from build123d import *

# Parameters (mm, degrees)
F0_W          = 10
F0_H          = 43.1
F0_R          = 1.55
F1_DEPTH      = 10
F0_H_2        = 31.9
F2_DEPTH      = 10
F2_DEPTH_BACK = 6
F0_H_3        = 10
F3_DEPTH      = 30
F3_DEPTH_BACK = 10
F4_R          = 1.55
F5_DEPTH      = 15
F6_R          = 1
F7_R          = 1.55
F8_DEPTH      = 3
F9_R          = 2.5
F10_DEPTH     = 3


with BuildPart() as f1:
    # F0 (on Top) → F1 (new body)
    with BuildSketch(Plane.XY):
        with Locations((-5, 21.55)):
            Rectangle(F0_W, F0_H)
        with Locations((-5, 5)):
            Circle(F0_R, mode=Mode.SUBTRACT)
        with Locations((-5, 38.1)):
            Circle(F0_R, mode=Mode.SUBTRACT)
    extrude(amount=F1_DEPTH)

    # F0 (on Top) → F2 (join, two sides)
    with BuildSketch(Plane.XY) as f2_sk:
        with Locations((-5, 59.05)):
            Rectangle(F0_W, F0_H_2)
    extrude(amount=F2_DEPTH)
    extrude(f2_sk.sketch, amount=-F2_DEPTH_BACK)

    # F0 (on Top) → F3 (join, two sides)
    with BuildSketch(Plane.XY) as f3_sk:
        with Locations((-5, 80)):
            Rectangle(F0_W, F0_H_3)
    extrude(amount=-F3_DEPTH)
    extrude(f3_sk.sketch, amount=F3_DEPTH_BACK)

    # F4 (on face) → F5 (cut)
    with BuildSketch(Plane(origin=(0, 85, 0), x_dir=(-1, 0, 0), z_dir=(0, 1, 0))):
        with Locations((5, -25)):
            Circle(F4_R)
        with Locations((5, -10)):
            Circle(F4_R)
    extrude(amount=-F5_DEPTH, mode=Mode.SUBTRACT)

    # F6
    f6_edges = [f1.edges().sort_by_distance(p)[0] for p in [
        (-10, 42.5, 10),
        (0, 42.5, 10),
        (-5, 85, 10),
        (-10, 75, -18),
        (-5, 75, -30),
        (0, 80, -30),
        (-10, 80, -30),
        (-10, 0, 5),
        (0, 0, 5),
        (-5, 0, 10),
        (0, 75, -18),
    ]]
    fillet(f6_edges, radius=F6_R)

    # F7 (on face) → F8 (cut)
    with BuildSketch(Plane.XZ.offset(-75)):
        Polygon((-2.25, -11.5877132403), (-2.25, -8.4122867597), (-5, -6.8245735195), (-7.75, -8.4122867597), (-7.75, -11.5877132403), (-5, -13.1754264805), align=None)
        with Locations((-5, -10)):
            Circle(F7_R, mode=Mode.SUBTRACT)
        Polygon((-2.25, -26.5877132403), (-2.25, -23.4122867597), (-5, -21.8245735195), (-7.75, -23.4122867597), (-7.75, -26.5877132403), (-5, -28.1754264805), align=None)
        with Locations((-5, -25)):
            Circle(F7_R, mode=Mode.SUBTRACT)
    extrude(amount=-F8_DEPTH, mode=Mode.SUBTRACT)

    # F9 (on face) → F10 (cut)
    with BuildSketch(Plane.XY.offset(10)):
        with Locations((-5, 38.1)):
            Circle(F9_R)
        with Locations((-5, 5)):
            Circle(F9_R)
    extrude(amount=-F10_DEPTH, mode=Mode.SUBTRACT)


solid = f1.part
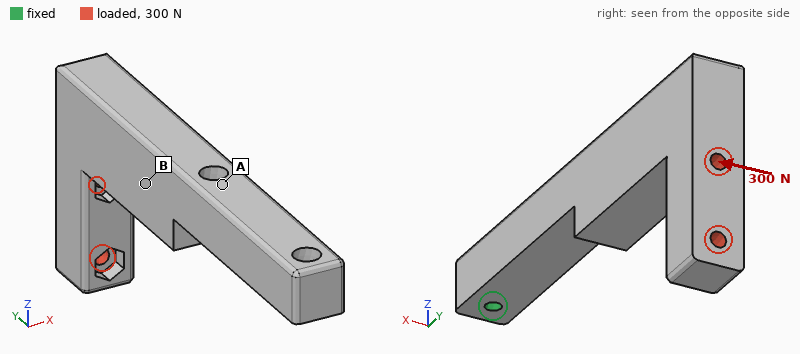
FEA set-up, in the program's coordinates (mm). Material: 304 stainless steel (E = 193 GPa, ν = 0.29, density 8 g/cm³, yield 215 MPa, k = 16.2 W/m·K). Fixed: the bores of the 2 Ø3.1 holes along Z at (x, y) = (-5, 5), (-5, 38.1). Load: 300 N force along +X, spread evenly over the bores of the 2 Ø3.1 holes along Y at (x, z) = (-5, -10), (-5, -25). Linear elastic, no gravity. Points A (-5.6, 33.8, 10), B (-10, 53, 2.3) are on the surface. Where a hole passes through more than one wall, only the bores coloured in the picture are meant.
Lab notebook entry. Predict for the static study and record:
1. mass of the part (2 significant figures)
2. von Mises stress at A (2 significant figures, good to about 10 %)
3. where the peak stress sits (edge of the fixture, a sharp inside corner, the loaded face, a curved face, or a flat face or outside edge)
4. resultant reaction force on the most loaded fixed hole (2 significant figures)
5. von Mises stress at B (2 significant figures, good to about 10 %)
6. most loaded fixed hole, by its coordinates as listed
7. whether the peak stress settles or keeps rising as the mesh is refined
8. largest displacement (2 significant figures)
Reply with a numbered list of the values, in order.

1. 100 g
2. 20 MPa
3. edge of the fixture
4. 510 N
5. 45 MPa
6. (-5, 38.1)
7. keeps rising
8. 0.12 mm
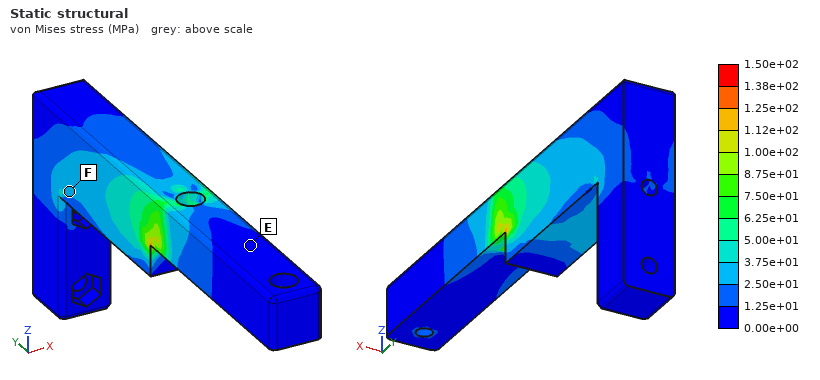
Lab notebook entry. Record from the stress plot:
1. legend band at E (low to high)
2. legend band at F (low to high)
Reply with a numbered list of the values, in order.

1. 0.00e+00 to 1.25e+01 MPa
2. 2.50e+01 to 3.75e+01 MPa
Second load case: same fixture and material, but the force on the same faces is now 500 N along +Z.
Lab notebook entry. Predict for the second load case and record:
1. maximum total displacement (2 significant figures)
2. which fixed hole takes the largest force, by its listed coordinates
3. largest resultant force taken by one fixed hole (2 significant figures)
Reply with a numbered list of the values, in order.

1. 0.11 mm
2. (-5, 38.1)
3. 780 N
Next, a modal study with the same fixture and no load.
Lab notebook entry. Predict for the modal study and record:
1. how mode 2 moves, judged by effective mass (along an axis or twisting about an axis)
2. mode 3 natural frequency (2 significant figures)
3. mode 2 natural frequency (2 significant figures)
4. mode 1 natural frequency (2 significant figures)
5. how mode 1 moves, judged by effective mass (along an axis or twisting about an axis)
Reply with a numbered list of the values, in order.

1. along Z
2. 4500 Hz
3. 2000 Hz
4. 1700 Hz
5. along X
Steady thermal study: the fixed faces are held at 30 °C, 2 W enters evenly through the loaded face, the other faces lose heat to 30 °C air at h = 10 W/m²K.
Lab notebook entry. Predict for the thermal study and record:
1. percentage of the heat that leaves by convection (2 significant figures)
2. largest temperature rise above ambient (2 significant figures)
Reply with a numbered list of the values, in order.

1. 39 %
2. 43 K
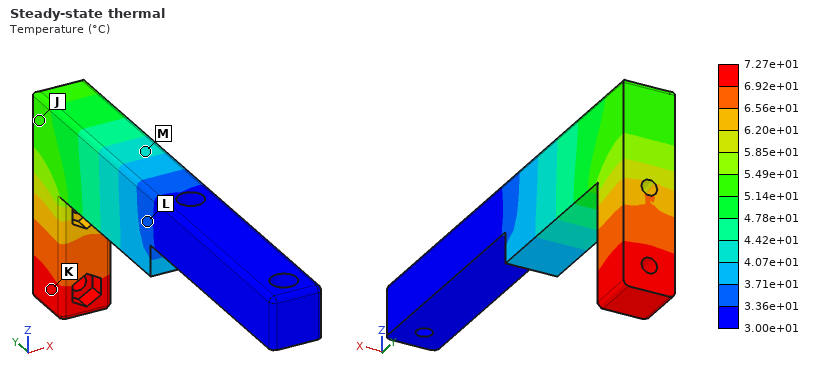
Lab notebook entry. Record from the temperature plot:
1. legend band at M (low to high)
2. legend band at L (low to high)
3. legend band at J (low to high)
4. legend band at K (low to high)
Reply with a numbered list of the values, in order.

1. 4.07e+01 to 4.42e+01 °C
2. 3.36e+01 to 3.71e+01 °C
3. 5.14e+01 to 5.49e+01 °C
4. 6.92e+01 to 7.27e+01 °C
